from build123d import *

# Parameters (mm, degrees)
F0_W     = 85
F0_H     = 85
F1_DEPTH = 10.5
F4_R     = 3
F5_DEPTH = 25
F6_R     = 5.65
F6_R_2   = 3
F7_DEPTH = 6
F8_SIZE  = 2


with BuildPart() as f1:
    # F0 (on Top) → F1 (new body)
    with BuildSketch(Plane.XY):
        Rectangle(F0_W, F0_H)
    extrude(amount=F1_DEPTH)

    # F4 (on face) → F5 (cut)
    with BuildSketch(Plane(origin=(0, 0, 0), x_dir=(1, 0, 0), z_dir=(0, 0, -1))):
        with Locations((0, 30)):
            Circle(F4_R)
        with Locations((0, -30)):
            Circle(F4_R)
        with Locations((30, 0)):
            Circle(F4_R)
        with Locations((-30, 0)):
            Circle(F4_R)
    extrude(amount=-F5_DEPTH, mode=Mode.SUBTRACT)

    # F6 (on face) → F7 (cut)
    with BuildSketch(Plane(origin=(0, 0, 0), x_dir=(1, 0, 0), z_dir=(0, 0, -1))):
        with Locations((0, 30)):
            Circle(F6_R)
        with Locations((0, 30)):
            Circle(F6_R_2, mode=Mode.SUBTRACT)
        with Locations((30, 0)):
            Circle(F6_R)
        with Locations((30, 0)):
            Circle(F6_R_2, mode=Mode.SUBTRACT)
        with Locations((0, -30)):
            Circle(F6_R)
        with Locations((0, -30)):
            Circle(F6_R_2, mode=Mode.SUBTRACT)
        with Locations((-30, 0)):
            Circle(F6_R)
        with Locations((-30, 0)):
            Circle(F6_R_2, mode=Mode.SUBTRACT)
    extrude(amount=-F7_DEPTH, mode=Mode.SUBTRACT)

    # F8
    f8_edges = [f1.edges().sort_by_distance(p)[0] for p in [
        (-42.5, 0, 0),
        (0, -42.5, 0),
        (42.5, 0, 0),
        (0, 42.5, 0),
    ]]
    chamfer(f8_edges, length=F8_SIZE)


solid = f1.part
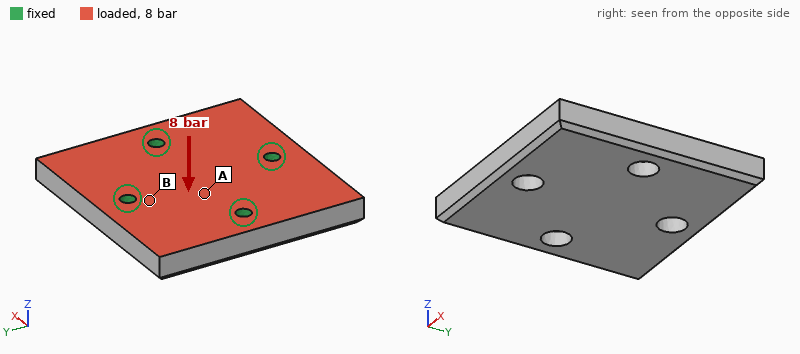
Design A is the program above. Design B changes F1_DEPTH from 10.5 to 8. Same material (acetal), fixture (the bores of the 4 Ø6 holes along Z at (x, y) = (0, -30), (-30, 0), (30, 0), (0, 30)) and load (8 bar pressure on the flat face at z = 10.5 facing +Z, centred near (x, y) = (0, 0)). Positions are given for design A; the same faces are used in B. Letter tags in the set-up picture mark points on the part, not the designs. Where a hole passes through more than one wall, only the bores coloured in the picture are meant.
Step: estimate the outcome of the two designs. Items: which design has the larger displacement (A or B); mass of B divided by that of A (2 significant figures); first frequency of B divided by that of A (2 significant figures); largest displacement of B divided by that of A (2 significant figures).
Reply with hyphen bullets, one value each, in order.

- B
- 0.75
- 0.76
- 2.2
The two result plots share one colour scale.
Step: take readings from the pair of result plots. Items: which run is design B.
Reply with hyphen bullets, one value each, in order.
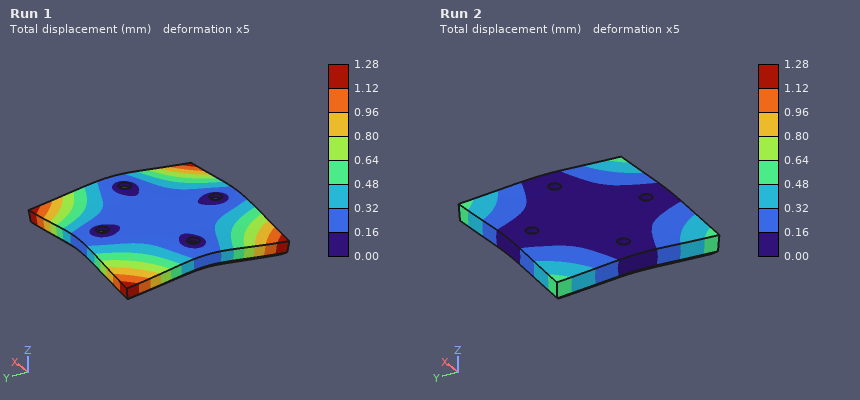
- Run 1
